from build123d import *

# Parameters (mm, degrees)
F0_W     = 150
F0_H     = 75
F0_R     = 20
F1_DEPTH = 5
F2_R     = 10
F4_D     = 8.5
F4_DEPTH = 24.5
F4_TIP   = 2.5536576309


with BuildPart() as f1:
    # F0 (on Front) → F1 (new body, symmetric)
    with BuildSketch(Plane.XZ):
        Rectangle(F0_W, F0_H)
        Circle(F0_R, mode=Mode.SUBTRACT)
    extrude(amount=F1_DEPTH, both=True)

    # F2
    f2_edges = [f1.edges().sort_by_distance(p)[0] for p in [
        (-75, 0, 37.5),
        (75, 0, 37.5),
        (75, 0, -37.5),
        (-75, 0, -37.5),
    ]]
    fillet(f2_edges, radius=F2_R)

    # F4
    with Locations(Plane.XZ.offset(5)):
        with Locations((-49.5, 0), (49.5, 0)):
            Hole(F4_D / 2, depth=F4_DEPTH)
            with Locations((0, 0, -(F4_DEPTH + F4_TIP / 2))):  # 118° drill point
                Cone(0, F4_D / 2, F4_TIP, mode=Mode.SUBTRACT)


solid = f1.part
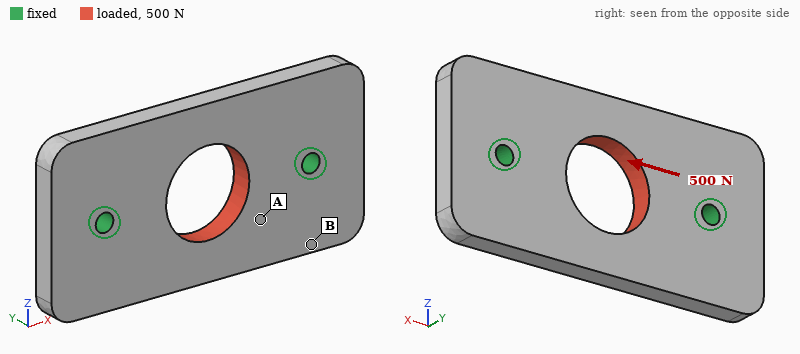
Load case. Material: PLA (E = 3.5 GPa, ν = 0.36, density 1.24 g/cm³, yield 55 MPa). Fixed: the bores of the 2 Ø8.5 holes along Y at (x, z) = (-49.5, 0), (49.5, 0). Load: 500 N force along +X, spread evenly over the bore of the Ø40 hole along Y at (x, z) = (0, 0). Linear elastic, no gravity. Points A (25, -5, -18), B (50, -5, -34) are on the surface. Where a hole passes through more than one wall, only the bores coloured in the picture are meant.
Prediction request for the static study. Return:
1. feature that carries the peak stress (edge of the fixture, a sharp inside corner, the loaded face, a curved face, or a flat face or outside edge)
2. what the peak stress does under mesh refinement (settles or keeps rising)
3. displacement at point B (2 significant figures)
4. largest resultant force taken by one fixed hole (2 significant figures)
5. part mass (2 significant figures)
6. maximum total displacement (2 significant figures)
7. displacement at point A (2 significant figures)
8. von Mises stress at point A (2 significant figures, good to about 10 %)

edge of the fixture
keeps rising
5.5 µm
250 N
120 g
9.1 µm
6.1 µm
0.50 MPa
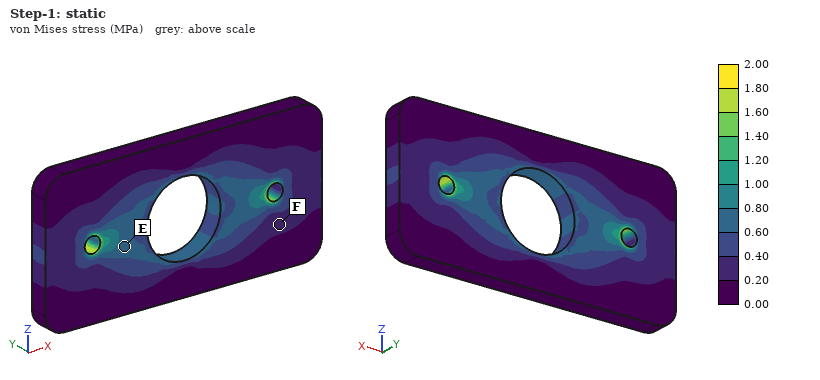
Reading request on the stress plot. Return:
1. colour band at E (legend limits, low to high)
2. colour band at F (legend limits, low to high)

0.60 to 0.80 MPa
0.20 to 0.40 MPa
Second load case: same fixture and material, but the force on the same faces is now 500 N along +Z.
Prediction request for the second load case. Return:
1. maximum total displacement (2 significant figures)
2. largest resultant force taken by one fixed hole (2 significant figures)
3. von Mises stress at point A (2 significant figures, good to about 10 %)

21 µm
250 N
0.72 MPa
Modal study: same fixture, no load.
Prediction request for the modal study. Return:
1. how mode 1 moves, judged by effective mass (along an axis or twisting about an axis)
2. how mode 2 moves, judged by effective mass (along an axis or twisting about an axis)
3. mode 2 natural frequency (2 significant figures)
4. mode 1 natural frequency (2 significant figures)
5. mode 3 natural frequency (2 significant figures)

twisting about X
along Y
1300 Hz
1100 Hz
1700 Hz
